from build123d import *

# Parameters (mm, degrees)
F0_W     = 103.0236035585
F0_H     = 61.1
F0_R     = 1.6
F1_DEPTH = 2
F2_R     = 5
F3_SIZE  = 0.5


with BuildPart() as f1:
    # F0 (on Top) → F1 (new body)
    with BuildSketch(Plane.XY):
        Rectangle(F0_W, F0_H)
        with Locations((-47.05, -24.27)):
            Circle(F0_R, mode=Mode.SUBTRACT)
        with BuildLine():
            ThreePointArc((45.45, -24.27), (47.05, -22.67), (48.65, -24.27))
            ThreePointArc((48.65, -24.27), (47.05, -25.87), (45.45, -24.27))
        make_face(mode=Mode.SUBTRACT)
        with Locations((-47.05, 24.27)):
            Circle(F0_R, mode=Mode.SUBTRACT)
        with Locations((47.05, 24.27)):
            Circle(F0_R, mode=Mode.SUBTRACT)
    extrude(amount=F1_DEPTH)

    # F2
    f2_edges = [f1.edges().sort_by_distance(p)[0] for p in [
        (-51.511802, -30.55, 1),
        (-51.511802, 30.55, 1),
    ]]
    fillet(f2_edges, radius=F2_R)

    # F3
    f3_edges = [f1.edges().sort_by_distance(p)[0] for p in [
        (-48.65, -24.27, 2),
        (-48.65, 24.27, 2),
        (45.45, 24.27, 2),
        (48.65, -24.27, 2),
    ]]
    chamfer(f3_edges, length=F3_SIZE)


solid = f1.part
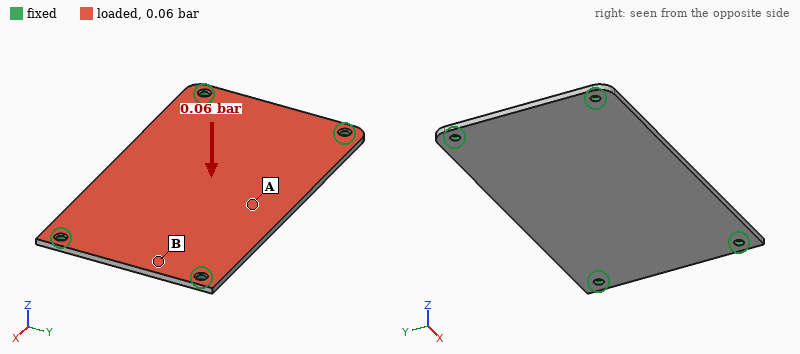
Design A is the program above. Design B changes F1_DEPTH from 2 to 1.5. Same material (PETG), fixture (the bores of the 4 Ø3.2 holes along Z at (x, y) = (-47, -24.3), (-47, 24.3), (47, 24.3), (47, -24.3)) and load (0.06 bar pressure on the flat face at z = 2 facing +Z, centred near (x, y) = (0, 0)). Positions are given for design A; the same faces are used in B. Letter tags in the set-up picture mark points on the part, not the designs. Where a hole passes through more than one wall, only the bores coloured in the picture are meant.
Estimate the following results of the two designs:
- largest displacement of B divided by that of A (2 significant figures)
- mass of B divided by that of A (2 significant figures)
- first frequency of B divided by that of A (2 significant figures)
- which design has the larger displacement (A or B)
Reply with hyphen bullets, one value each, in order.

- 2.3
- 0.75
- 0.75
- B
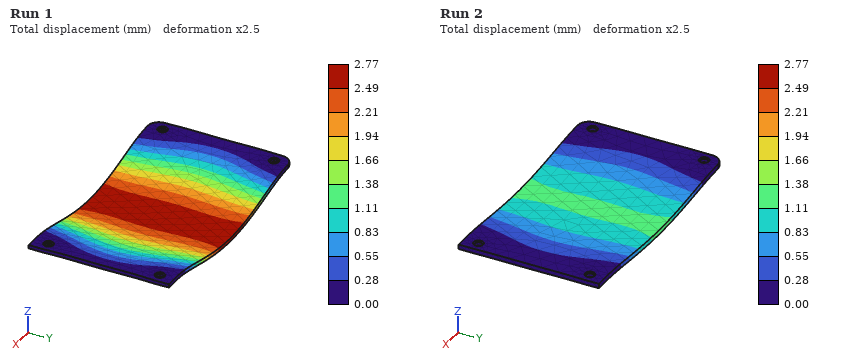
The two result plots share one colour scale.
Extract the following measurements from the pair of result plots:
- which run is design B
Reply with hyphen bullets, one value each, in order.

- Run 1
